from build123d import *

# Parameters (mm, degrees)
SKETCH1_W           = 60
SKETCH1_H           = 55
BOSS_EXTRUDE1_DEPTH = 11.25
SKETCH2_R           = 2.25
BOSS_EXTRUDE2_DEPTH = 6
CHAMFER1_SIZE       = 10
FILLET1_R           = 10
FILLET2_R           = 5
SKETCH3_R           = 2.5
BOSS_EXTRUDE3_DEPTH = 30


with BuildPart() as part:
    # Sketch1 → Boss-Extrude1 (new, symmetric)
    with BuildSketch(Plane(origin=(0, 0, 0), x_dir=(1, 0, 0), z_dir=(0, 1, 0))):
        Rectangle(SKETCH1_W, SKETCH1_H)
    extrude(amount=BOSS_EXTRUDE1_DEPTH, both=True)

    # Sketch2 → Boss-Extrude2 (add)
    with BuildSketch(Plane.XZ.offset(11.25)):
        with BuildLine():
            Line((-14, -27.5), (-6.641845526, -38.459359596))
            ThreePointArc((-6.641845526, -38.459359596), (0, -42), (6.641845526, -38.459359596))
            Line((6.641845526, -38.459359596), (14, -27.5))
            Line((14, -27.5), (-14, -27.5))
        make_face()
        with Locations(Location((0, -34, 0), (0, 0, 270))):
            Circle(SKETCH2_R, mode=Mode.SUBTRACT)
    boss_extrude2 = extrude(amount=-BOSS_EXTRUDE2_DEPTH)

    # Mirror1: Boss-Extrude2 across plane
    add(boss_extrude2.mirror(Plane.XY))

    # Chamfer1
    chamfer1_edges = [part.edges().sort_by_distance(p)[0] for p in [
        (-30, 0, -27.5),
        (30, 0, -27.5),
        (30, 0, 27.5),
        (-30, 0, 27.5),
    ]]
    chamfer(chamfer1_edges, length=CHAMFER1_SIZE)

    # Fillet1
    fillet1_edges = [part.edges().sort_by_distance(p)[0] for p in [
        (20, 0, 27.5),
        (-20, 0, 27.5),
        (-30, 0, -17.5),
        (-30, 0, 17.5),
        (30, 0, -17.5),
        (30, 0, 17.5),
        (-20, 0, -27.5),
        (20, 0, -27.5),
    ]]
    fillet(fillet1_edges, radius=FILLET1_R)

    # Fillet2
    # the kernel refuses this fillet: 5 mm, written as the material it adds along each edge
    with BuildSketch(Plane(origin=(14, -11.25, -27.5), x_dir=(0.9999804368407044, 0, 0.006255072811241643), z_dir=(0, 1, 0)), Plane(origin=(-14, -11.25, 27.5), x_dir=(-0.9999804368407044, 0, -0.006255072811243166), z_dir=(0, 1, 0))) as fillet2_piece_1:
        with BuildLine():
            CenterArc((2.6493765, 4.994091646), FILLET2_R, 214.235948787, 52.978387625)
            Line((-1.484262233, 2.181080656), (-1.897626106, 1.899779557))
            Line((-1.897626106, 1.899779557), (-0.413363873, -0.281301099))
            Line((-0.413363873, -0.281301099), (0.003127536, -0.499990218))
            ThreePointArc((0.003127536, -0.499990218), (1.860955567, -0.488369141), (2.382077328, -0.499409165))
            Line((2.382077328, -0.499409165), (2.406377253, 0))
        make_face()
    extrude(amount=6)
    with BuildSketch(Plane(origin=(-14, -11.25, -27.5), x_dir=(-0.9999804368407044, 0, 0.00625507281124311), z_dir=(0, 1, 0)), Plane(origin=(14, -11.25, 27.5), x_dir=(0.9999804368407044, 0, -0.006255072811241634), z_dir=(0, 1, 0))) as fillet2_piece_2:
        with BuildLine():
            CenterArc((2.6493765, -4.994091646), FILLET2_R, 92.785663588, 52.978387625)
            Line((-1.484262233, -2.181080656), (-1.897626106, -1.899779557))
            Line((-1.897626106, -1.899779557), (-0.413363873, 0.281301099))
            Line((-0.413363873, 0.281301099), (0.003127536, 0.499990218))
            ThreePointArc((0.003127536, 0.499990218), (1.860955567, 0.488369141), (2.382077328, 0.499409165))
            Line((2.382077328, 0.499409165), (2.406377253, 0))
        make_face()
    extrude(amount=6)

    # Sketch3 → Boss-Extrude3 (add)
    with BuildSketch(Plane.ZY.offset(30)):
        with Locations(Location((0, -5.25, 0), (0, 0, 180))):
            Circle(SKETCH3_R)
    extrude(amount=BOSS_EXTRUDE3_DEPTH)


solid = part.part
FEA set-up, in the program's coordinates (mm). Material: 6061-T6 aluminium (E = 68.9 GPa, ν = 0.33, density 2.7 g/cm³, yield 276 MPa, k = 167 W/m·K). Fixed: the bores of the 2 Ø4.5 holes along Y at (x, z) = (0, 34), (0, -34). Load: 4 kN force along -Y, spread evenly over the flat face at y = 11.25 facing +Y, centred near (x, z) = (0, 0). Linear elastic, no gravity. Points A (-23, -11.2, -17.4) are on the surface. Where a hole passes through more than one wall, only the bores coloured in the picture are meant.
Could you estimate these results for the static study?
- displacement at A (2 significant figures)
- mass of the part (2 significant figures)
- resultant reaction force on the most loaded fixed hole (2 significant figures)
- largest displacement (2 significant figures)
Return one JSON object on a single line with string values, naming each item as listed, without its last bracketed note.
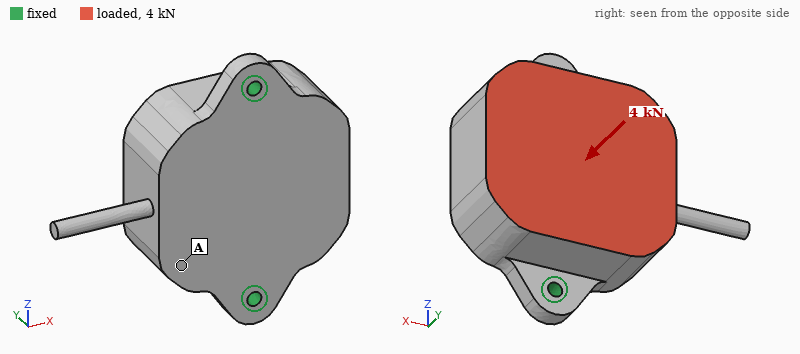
{"displacement at A": "17 µm", "mass of the part": "200 g", "resultant reaction force on the most loaded fixed hole": "2.3 kN", "largest displacement": "22 µm"}
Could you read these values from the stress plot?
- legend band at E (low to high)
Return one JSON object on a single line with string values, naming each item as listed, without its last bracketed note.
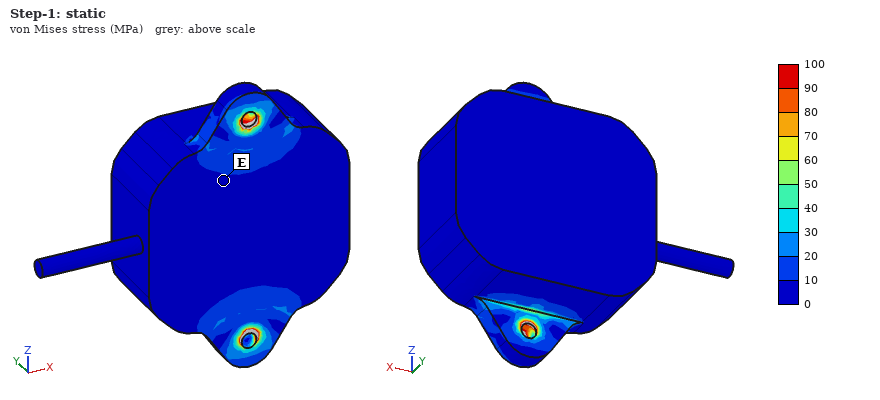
{"legend band at E": "0 to 10 MPa"}
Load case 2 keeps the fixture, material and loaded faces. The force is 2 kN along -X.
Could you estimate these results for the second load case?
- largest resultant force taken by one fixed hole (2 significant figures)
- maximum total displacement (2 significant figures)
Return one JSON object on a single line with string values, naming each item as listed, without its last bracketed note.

{"largest resultant force taken by one fixed hole": "1.0 kN", "maximum total displacement": "0.24 mm"}
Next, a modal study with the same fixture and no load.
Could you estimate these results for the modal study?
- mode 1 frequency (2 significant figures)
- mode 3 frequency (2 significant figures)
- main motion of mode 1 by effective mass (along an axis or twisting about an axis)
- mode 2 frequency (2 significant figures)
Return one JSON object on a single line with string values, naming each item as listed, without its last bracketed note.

{"mode 1 frequency": "1800 Hz", "mode 3 frequency": "3700 Hz", "main motion of mode 1 by effective mass": "along X", "mode 2 frequency": "3600 Hz"}
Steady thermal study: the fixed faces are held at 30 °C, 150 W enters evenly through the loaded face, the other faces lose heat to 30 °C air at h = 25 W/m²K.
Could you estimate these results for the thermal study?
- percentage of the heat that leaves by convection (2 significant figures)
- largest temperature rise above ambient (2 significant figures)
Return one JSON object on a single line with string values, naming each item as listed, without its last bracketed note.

{"percentage of the heat that leaves by convection": "5.6 %", "largest temperature rise above ambient": "46 K"}
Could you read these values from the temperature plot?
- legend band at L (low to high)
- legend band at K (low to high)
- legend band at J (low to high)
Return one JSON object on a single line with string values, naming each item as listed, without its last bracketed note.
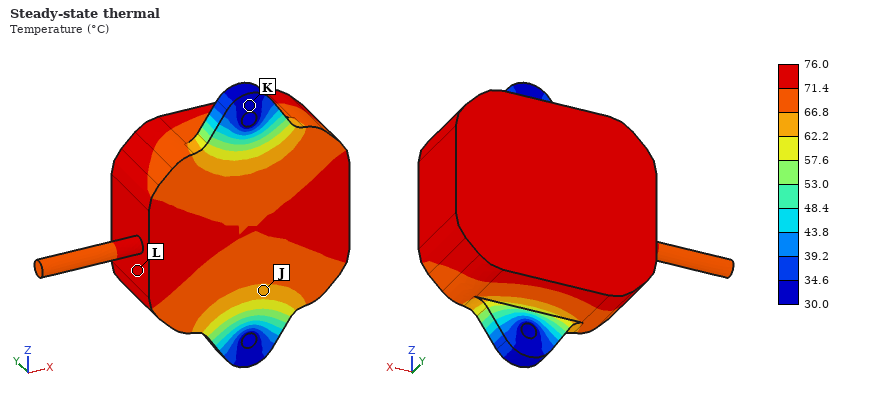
{"legend band at L": "71.4 to 76.0 °C", "legend band at K": "30.0 to 34.6 °C", "legend band at J": "62.2 to 66.8 °C"}
